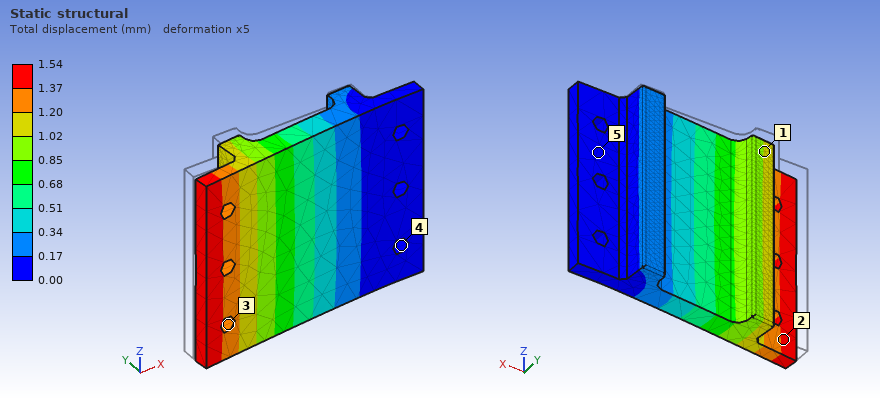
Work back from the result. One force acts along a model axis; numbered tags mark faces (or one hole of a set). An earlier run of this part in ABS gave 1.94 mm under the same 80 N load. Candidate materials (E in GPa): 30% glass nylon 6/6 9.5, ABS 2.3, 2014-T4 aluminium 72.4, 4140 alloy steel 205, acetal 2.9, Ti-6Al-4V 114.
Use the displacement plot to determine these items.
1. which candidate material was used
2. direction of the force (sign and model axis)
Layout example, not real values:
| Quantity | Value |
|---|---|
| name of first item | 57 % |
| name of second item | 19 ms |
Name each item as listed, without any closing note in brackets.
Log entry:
| Quantity | Value |
|---|---|
| which candidate material was used | acetal |
| direction of the force | -Y |
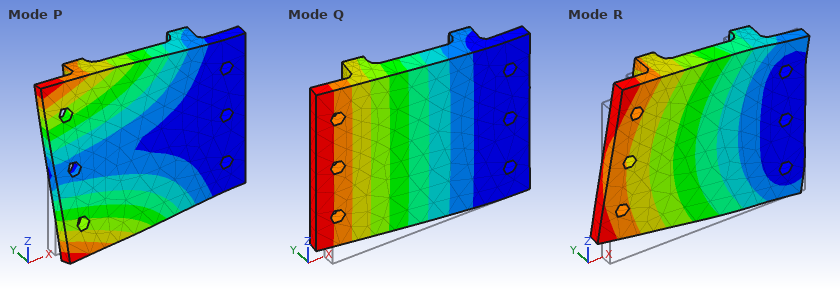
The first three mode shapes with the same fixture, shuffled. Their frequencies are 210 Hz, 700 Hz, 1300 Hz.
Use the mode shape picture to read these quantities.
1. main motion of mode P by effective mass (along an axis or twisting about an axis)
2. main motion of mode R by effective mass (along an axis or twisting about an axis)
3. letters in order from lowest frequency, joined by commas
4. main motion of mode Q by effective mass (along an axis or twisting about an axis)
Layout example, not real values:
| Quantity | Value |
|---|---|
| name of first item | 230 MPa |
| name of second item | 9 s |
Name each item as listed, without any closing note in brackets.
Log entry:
| Quantity | Value |
|---|---|
| main motion of mode P by effective mass | twisting about X |
| main motion of mode R by effective mass | along Z |
| letters in order from lowest frequency, joined by commas | Q, P, R |
| main motion of mode Q by effective mass | along Y |
